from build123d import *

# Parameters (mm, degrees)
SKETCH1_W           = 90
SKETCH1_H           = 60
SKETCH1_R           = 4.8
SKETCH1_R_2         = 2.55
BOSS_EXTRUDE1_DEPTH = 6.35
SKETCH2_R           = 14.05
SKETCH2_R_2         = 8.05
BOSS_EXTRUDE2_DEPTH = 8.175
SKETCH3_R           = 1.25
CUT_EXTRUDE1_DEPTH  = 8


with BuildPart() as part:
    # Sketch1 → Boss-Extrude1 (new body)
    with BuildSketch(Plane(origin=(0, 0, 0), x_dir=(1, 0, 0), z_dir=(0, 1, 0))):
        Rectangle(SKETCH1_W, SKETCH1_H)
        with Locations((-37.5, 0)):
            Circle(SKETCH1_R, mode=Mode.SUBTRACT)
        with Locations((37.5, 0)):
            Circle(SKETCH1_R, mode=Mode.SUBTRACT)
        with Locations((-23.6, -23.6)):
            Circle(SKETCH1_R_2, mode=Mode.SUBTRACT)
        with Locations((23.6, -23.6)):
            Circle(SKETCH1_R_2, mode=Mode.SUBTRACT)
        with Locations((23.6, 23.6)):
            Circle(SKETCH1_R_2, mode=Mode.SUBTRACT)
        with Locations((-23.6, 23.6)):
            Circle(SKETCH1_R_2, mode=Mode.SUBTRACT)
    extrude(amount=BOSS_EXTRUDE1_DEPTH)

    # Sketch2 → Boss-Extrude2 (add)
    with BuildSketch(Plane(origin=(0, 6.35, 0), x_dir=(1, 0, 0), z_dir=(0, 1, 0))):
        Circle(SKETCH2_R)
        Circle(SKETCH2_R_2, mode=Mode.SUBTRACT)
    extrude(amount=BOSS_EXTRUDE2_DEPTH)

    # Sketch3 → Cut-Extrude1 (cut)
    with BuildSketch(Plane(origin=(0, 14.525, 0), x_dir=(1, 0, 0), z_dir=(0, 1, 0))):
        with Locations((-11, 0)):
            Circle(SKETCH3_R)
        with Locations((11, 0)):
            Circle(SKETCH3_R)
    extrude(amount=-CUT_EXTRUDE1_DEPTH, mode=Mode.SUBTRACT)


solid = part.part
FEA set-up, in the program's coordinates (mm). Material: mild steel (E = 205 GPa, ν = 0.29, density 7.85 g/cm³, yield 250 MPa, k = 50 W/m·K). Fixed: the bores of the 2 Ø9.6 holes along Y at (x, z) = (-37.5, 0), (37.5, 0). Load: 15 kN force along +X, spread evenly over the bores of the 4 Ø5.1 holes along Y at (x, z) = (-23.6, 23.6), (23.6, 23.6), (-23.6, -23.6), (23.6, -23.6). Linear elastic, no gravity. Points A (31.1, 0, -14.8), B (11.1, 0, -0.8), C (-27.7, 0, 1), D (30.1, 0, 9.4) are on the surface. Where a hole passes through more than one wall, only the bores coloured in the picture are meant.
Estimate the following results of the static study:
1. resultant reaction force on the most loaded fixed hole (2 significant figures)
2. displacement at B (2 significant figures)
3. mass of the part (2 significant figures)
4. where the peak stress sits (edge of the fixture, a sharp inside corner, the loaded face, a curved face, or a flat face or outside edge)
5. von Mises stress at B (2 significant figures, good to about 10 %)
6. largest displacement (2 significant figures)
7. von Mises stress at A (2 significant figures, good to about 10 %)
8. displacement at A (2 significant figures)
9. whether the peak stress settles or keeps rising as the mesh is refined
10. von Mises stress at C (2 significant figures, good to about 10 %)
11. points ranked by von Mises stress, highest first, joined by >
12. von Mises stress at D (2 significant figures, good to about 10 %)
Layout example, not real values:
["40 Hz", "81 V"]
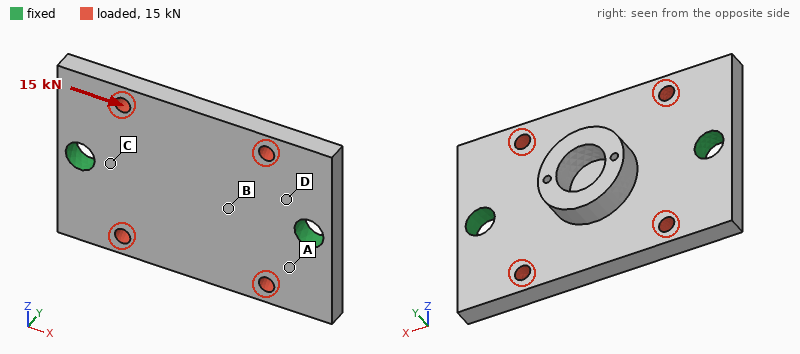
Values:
["7.5 kN", "3.5 µm", "280 g", "edge of the fixture", "17 MPa", "8.0 µm", "28 MPa", "4.0 µm", "keeps rising", "47 MPa", "C > D > A > B", "36 MPa"]
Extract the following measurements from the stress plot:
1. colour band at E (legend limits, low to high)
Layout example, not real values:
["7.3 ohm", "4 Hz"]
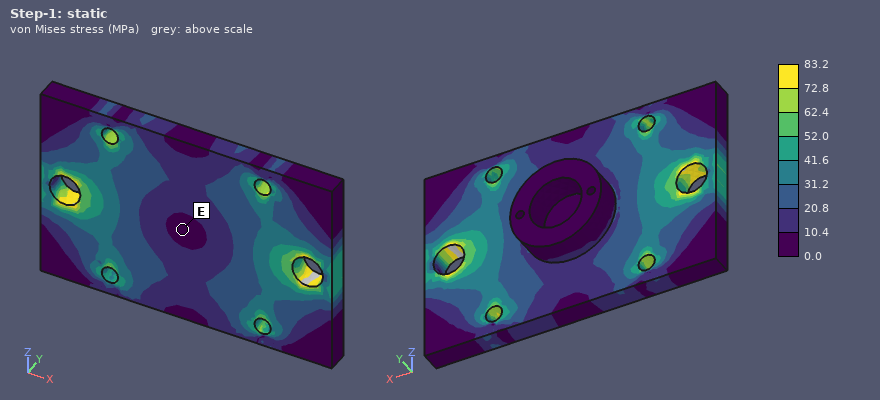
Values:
["0.0 to 10.4 MPa"]
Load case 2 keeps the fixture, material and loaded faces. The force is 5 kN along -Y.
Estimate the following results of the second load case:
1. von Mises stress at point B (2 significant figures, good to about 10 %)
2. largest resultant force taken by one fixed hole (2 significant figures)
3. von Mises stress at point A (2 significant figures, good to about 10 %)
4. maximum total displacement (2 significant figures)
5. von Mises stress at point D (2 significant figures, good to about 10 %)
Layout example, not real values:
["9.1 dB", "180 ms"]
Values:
["49 MPa", "2.5 kN", "33 MPa", "39 µm", "56 MPa"]
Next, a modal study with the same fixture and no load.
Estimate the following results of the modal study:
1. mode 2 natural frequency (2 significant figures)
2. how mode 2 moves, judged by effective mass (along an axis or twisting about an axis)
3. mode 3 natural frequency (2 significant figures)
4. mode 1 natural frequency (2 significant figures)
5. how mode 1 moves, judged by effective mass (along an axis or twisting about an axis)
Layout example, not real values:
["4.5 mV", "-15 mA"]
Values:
["4800 Hz", "along Y", "8100 Hz", "3900 Hz", "twisting about X"]
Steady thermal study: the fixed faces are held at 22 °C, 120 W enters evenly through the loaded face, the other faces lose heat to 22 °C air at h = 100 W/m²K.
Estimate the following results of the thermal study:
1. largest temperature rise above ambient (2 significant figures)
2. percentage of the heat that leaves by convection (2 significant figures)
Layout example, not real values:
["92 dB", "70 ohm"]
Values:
["77 K", "42 %"]
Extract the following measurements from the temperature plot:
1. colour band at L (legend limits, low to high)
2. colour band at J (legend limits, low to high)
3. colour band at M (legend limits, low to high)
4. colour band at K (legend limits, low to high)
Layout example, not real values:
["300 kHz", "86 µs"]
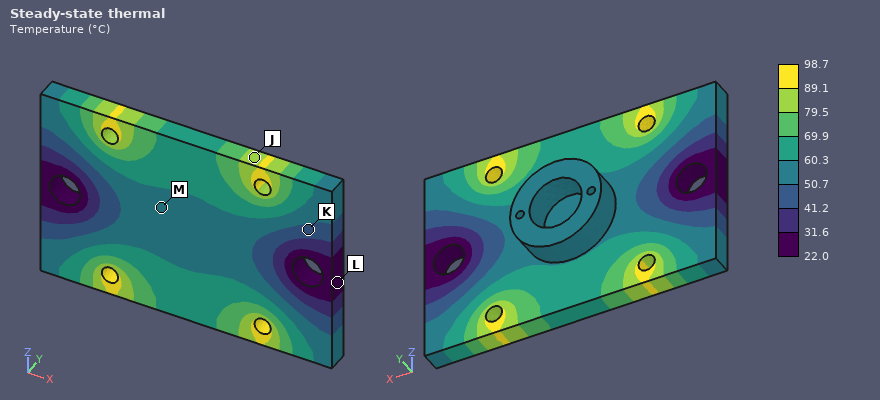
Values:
["22.0 to 31.6 °C", "79.5 to 89.1 °C", "50.7 to 60.3 °C", "41.2 to 50.7 °C"]
